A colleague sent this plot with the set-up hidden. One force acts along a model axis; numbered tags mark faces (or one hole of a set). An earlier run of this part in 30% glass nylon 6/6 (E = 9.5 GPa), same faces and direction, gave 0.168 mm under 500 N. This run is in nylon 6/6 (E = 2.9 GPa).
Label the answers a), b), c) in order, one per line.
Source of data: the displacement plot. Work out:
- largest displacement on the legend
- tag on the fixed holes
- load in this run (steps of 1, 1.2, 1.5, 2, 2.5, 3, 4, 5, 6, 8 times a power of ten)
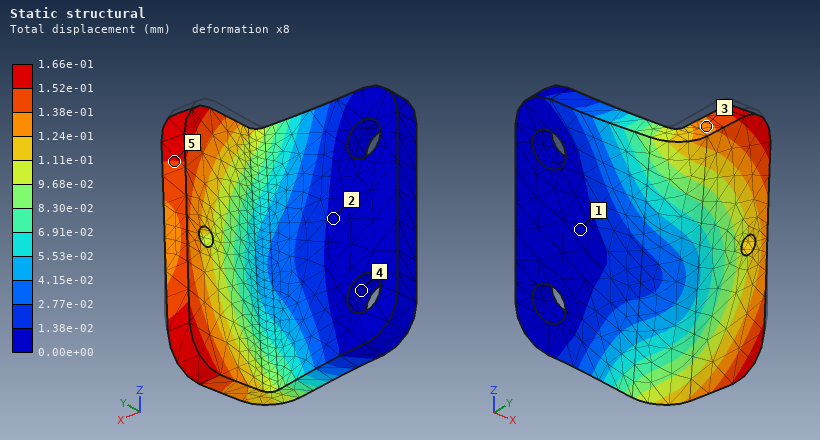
a) 1.66e-01 mm
b) 4
c) 150 N
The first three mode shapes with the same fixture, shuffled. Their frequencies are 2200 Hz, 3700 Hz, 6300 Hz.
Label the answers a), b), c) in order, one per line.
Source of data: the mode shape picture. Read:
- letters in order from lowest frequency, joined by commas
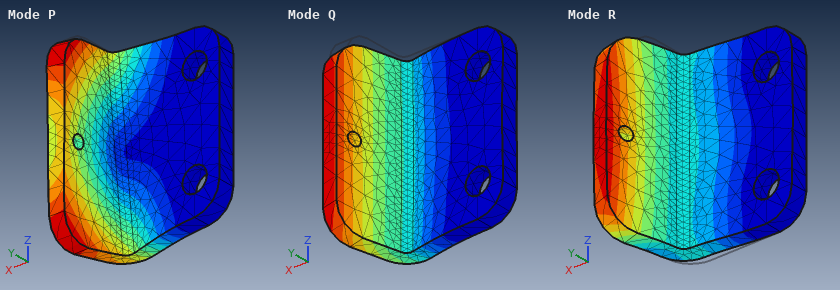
a) Q, P, R
